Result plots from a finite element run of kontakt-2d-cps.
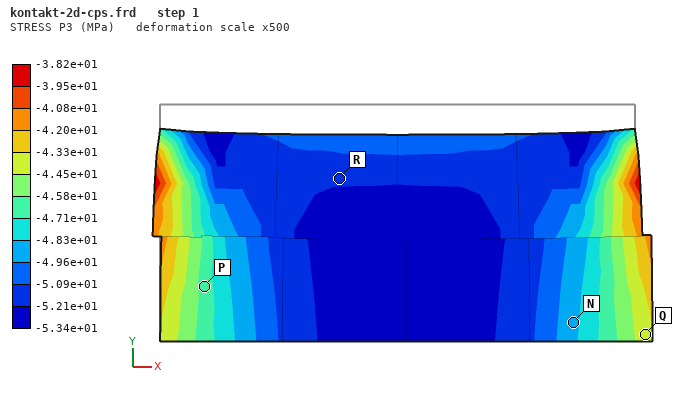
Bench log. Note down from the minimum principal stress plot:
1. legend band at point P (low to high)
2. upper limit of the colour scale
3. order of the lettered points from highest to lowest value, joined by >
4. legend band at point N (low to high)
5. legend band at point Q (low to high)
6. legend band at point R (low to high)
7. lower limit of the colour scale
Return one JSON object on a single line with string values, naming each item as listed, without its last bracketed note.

{"legend band at point P": "-4.71e+01 to -4.58e+01 MPa", "upper limit of the colour scale": "-3.82e+01 MPa", "order of the lettered points from highest to lowest value, joined by >": "Q > P > N > R", "legend band at point N": "-4.96e+01 to -4.83e+01 MPa", "legend band at point Q": "-4.45e+01 to -4.33e+01 MPa", "legend band at point R": "-5.21e+01 to -5.09e+01 MPa", "lower limit of the colour scale": "-5.34e+01 MPa"}
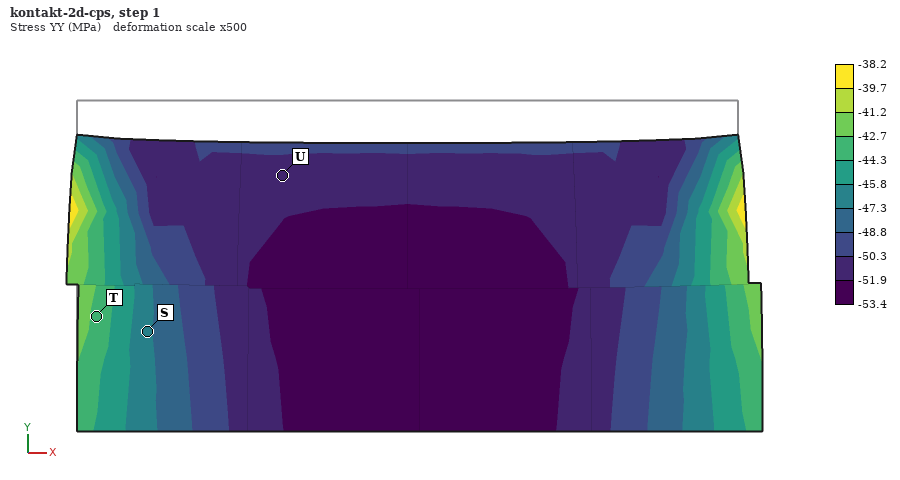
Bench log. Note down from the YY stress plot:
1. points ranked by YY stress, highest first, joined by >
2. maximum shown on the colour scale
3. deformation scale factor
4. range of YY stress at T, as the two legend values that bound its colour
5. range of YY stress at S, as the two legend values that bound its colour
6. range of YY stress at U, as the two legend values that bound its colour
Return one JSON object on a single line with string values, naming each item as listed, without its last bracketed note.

{"points ranked by YY stress, highest first, joined by >": "T > S > U", "maximum shown on the colour scale": "-38.2 MPa", "deformation scale factor": "500", "range of YY stress at T, as the two legend values that bound its colour": "-44.3 to -42.7 MPa", "range of YY stress at S, as the two legend values that bound its colour": "-47.3 to -45.8 MPa", "range of YY stress at U, as the two legend values that bound its colour": "-51.9 to -50.3 MPa"}
